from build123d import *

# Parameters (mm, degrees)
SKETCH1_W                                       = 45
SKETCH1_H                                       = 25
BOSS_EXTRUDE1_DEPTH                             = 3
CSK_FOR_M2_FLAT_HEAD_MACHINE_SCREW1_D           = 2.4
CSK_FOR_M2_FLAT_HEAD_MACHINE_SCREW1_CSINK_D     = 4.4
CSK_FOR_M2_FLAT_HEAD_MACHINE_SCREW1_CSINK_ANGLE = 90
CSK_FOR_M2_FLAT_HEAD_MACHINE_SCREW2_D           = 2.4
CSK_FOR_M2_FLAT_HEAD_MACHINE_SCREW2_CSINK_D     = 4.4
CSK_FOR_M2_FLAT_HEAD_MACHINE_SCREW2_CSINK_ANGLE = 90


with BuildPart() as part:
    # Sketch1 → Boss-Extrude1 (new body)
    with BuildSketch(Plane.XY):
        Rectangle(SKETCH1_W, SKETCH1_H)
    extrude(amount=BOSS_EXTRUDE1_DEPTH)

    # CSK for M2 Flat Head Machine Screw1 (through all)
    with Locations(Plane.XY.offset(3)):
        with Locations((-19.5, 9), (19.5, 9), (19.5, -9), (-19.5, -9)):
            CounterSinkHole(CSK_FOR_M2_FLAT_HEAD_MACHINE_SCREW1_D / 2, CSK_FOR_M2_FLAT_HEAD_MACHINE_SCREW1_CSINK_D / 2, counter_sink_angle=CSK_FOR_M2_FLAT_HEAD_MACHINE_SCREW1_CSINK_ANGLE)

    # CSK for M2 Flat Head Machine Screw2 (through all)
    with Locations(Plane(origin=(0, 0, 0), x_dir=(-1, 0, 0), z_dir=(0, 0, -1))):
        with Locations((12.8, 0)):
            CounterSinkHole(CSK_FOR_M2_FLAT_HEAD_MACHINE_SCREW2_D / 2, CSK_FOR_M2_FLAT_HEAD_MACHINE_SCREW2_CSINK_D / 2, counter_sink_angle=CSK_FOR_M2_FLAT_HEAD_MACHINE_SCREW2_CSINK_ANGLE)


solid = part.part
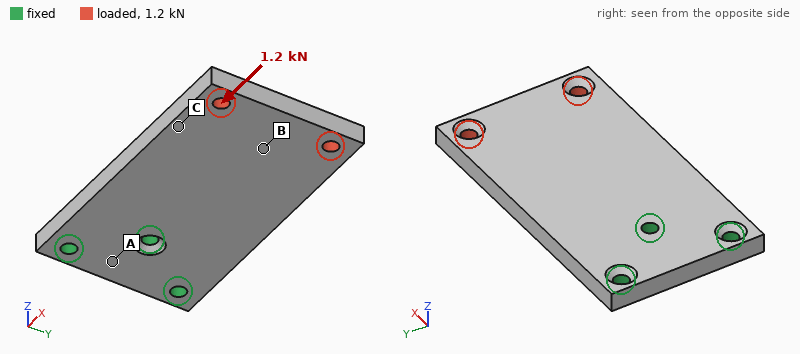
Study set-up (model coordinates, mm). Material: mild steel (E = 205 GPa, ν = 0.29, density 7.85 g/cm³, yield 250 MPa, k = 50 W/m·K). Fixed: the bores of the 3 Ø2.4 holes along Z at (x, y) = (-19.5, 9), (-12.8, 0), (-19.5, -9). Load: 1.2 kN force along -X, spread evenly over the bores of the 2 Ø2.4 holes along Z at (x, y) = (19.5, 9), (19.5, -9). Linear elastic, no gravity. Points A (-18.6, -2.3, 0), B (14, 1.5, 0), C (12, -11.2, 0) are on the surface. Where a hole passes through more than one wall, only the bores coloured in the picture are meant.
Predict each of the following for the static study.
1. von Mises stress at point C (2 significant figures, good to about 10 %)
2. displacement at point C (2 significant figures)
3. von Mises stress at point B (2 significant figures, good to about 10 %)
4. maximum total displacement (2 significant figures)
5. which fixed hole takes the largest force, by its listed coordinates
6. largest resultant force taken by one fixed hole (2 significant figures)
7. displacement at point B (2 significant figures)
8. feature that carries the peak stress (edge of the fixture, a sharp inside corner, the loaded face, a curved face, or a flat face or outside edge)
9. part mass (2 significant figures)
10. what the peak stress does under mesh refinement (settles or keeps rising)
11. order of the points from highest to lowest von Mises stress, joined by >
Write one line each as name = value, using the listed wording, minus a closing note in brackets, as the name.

von Mises stress at point C = 40 MPa
displacement at point C = 20 µm
von Mises stress at point B = 21 MPa
maximum total displacement = 38 µm
which fixed hole takes the largest force, by its listed coordinates = (-12.8, 0)
largest resultant force taken by one fixed hole = 560 N
displacement at point B = 23 µm
feature that carries the peak stress = edge of the fixture
part mass = 26 g
what the peak stress does under mesh refinement = keeps rising
order of the points from highest to lowest von Mises stress, joined by > = C > B > A
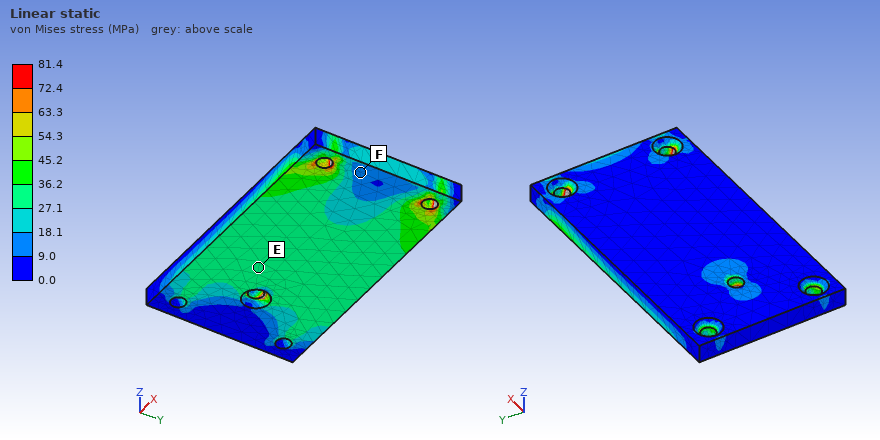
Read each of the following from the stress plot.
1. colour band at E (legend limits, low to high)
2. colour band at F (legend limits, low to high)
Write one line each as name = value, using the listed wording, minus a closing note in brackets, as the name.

colour band at E = 27.1 to 36.2 MPa
colour band at F = 9.0 to 18.1 MPa
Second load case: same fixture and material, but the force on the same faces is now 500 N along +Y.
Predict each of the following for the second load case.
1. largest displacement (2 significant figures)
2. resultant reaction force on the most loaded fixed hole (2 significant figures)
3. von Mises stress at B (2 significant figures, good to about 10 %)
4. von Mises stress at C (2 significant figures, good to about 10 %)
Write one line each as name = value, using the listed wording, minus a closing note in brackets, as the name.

largest displacement = 21 µm
resultant reaction force on the most loaded fixed hole = 790 N
von Mises stress at B = 21 MPa
von Mises stress at C = 14 MPa
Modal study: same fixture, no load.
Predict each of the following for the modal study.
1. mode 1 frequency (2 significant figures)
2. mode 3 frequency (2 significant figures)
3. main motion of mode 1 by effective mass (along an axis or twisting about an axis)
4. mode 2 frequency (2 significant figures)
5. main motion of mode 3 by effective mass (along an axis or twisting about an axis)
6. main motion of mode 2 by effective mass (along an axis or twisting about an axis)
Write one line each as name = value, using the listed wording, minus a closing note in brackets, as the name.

mode 1 frequency = 1800 Hz
mode 3 frequency = 9900 Hz
main motion of mode 1 by effective mass = along Z
mode 2 frequency = 5200 Hz
main motion of mode 3 by effective mass = along Y
main motion of mode 2 by effective mass = twisting about X
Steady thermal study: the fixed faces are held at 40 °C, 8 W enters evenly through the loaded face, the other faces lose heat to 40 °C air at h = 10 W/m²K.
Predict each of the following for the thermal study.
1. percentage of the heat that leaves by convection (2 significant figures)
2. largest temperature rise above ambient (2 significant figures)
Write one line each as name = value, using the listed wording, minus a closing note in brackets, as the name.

percentage of the heat that leaves by convection = 11 %
largest temperature rise above ambient = 80 K
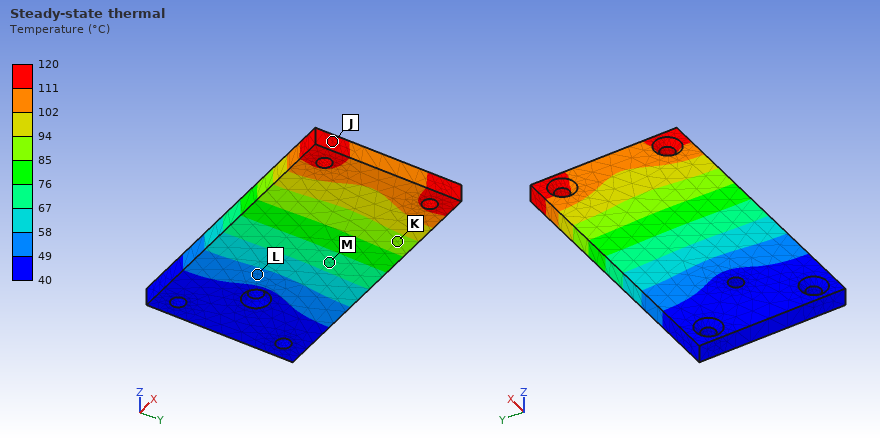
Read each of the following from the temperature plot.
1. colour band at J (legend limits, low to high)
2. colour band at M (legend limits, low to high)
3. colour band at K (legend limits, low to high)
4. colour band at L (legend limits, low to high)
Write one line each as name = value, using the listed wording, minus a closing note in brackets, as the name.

colour band at J = 111 to 120 °C
colour band at M = 67 to 76 °C
colour band at K = 85 to 94 °C
colour band at L = 49 to 58 °C
